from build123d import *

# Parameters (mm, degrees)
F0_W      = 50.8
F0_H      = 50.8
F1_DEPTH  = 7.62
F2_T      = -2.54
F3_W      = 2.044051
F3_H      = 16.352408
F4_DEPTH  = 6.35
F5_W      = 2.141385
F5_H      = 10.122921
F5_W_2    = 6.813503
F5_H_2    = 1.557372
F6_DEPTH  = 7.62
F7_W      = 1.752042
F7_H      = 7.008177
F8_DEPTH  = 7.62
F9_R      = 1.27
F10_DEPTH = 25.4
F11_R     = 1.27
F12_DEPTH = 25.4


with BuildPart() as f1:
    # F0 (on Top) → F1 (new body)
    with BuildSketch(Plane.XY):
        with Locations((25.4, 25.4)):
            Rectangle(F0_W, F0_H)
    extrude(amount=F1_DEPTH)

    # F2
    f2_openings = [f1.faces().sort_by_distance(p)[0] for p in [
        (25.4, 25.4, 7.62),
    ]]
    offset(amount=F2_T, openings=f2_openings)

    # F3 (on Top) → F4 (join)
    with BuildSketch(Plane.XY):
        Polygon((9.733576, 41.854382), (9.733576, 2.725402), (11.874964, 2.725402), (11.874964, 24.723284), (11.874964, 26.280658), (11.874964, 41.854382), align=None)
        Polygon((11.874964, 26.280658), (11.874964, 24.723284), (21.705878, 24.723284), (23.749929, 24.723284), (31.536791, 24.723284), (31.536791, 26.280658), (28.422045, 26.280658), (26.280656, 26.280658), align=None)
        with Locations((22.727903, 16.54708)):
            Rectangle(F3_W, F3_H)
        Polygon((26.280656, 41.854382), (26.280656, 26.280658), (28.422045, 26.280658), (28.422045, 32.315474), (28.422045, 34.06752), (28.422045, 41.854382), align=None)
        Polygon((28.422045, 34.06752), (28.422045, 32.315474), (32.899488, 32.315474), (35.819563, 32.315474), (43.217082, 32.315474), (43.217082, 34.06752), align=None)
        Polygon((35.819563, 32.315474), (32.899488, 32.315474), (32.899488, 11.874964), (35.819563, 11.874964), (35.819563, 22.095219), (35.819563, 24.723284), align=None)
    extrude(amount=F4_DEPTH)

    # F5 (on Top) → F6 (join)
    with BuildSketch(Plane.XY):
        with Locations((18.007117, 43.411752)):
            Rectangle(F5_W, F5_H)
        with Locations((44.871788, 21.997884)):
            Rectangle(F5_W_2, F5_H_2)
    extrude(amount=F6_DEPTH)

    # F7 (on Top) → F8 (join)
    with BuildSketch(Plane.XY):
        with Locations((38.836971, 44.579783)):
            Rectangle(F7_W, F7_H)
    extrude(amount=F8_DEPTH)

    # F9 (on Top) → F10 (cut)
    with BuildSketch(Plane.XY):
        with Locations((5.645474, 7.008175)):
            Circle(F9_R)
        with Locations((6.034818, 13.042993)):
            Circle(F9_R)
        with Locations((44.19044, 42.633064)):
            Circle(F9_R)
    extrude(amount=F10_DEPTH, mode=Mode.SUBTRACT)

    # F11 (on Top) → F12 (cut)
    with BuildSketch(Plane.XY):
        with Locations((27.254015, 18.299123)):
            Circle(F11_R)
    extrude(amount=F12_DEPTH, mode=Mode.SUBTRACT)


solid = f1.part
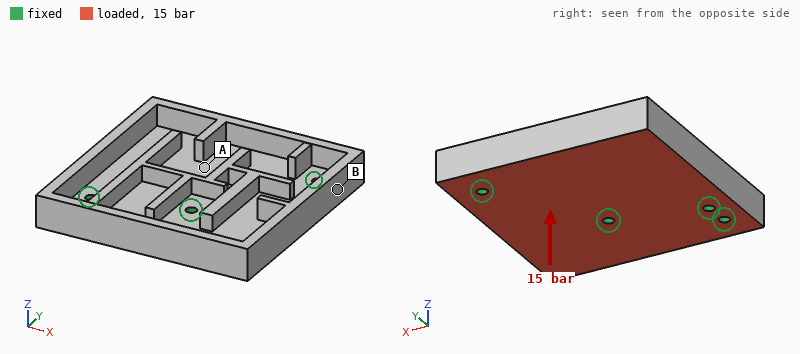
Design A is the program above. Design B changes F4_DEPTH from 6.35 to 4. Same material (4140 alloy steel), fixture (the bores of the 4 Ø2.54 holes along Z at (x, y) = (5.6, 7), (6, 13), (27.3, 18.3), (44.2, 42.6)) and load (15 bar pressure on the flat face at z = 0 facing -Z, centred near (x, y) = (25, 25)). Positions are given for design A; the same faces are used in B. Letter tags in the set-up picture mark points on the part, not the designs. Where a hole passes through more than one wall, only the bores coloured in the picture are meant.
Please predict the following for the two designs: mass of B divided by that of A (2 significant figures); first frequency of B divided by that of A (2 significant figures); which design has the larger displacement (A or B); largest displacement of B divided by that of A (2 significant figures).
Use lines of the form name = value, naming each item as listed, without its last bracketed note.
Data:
mass of B divided by that of A = 0.94
first frequency of B divided by that of A = 0.96
which design has the larger displacement = B
largest displacement of B divided by that of A = 1.2
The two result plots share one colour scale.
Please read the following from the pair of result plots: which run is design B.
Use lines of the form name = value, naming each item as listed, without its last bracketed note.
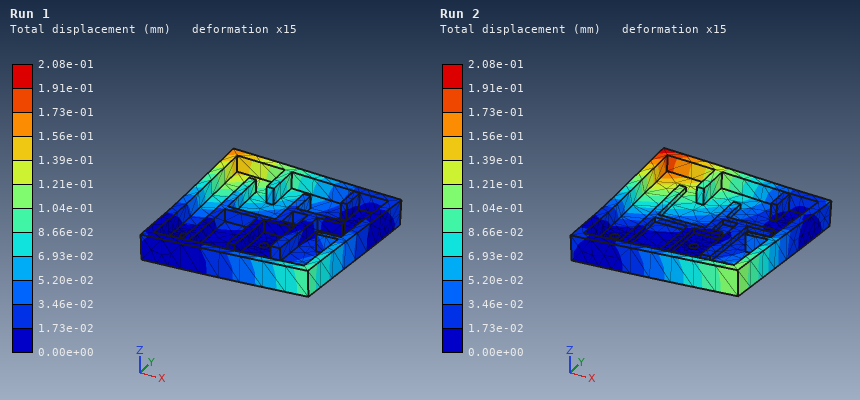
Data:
which run is design B = Run 2
